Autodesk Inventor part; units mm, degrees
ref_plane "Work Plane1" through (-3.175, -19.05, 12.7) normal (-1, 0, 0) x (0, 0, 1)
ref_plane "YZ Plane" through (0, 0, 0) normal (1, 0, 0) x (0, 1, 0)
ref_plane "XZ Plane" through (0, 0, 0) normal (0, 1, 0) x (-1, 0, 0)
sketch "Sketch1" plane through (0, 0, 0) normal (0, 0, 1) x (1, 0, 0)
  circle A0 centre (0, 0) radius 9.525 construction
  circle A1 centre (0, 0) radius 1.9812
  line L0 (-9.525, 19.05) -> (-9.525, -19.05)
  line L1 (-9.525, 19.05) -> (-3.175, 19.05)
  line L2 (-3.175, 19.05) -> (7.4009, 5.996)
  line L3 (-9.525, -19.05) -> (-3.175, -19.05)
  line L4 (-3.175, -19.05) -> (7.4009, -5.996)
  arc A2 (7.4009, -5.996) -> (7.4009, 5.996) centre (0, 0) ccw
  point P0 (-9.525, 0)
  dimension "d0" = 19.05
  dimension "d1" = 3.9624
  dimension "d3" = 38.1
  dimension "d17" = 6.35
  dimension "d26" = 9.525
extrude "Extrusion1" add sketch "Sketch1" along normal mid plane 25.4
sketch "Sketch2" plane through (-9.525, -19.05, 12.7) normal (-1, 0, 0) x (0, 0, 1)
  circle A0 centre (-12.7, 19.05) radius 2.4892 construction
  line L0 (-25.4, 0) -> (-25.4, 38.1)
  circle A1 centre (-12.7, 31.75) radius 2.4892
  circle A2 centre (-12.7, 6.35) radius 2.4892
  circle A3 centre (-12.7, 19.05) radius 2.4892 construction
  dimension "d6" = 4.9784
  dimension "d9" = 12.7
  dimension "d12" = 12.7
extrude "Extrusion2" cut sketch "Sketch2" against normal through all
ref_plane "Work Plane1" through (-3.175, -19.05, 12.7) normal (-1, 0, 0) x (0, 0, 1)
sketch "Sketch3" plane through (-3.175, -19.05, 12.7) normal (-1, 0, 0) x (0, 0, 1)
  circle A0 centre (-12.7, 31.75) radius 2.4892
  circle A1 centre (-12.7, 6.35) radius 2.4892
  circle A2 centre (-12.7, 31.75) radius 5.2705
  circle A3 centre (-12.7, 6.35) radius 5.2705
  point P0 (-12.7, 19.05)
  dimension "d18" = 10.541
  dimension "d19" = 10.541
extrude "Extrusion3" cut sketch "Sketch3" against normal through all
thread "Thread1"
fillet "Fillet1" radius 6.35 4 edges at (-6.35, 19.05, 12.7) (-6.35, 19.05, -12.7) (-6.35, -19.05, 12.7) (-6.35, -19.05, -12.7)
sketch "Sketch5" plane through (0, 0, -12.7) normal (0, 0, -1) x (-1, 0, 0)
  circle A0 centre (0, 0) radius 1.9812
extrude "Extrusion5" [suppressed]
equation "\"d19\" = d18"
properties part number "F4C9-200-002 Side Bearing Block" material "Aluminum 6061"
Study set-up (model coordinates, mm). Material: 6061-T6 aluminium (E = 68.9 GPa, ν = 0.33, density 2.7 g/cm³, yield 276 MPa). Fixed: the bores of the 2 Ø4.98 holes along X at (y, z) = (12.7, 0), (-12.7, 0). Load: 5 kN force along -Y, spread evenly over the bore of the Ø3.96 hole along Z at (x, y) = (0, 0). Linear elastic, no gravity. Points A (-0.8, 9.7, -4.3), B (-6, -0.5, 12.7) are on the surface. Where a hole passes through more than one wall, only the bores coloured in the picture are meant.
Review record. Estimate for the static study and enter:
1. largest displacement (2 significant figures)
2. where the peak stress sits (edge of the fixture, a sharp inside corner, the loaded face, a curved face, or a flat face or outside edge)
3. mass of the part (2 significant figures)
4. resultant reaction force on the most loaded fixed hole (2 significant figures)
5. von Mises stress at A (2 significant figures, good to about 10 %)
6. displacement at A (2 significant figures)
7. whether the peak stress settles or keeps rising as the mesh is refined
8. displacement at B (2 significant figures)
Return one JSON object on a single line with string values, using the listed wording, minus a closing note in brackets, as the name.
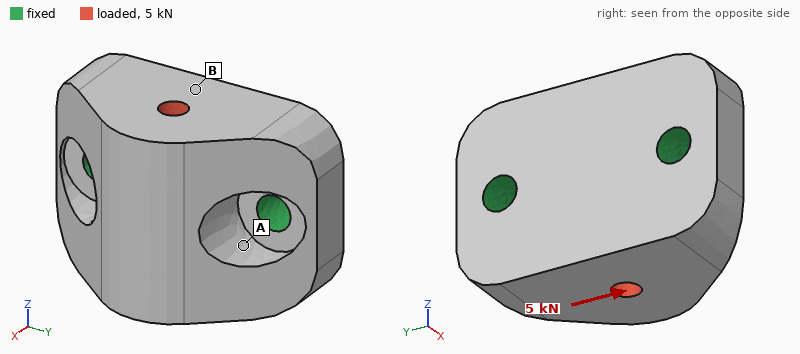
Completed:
{"largest displacement": "7.0 µm", "where the peak stress sits": "edge of the fixture", "mass of the part": "31 g", "resultant reaction force on the most loaded fixed hole": "2.8 kN", "von Mises stress at A": "16 MPa", "displacement at A": "4.6 µm", "whether the peak stress settles or keeps rising as the mesh is refined": "keeps rising", "displacement at B": "2.9 µm"}
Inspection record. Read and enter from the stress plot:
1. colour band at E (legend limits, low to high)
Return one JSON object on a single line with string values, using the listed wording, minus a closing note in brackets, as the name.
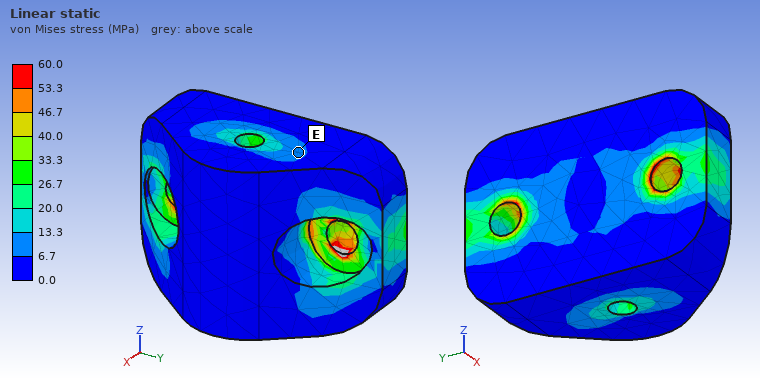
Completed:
{"colour band at E": "6.7 to 13.3 MPa"}
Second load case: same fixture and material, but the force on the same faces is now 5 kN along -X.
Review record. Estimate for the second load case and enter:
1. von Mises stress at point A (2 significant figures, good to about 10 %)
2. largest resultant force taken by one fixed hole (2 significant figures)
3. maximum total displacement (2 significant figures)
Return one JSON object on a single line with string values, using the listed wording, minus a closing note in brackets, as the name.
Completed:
{"von Mises stress at point A": "25 MPa", "largest resultant force taken by one fixed hole": "2.6 kN", "maximum total displacement": "10 µm"}
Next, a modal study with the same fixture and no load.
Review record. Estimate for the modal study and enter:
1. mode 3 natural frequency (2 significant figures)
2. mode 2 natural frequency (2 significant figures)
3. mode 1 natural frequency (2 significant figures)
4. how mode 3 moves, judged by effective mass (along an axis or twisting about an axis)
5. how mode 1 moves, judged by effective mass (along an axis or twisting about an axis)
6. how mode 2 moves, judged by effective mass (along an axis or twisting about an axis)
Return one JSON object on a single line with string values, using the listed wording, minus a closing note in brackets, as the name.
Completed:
{"mode 3 natural frequency": "29 kHz", "mode 2 natural frequency": "27 kHz", "mode 1 natural frequency": "13 kHz", "how mode 3 moves, judged by effective mass": "along Y", "how mode 1 moves, judged by effective mass": "along Z", "how mode 2 moves, judged by effective mass": "along X"}
